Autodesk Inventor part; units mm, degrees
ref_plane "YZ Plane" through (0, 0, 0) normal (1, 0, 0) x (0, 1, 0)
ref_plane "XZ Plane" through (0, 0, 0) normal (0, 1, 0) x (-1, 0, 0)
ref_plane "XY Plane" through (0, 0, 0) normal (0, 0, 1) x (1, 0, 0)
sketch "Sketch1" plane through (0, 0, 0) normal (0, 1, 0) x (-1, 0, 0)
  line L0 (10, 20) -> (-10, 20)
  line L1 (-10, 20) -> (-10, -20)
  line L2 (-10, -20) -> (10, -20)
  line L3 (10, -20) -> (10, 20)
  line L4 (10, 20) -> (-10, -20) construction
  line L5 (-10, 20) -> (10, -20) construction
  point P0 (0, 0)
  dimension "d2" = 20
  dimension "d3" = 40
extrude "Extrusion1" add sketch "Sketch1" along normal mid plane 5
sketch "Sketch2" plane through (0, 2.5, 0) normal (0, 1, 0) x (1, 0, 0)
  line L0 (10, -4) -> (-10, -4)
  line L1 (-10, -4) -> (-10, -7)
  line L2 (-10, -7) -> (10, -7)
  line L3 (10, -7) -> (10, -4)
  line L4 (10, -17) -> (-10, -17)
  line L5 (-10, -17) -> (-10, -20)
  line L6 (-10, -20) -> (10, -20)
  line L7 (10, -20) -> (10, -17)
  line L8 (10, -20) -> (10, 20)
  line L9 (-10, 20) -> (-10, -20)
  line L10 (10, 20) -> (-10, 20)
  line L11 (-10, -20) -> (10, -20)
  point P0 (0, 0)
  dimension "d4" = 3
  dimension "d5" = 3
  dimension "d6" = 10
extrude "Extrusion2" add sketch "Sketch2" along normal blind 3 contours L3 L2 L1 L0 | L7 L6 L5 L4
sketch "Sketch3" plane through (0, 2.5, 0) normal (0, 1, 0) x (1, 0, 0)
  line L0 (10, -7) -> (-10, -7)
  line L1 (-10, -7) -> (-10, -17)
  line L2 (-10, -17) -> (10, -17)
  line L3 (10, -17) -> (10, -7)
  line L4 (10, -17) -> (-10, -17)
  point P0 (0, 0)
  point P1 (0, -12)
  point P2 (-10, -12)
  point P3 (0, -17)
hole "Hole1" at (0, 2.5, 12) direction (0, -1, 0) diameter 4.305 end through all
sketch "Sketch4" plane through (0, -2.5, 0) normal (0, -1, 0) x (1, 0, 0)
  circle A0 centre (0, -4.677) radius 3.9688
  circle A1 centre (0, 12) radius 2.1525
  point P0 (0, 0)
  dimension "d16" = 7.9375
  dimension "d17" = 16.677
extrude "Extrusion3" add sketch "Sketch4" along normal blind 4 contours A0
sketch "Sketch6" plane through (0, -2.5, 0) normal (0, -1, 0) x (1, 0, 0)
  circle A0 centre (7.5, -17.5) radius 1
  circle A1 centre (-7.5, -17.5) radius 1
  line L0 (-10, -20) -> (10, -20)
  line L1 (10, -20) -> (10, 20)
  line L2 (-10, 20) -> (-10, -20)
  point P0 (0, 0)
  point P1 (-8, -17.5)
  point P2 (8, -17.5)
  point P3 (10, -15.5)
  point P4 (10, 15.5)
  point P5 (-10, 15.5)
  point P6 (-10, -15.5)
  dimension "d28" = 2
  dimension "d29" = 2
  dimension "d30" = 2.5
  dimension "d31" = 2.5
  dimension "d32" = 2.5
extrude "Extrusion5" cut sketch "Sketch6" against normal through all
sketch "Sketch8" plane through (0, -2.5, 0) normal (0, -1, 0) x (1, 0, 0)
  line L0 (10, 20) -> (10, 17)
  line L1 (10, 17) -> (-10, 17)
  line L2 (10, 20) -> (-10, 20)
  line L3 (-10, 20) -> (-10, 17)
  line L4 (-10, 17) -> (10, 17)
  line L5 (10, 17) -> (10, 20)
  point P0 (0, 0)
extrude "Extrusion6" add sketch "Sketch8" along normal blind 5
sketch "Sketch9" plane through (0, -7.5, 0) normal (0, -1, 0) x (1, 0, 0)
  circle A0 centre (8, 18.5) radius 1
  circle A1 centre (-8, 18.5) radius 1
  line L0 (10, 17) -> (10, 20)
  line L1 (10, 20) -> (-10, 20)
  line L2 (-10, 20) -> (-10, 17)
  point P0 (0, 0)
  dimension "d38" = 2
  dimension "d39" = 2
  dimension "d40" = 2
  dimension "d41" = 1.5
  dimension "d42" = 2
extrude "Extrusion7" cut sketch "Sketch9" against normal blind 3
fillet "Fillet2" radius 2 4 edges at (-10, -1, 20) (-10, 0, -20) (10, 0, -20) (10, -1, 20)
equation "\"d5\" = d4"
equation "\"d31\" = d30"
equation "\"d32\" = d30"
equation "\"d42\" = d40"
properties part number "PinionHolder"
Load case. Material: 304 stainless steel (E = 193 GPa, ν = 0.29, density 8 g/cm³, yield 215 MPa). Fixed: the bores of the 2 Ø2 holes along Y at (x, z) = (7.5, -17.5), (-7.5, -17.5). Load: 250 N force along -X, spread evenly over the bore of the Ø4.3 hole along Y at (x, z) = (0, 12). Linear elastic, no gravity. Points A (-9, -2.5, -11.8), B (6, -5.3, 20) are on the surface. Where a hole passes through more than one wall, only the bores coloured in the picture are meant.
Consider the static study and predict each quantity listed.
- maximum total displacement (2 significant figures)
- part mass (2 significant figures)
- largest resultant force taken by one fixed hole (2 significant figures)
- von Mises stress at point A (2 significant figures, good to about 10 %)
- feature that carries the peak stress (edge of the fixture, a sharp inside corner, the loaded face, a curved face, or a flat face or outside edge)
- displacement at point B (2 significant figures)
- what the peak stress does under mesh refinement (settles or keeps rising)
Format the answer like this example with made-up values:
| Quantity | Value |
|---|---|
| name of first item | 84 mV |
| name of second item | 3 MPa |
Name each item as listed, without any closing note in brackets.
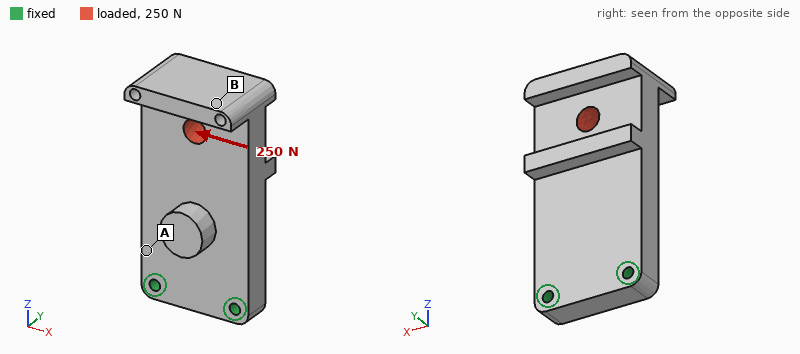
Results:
| Quantity | Value |
|---|---|
| maximum total displacement | 6.2 µm |
| part mass | 38 g |
| largest resultant force taken by one fixed hole | 490 N |
| von Mises stress at point A | 16 MPa |
| feature that carries the peak stress | edge of the fixture |
| displacement at point B | 6.0 µm |
| what the peak stress does under mesh refinement | keeps rising |
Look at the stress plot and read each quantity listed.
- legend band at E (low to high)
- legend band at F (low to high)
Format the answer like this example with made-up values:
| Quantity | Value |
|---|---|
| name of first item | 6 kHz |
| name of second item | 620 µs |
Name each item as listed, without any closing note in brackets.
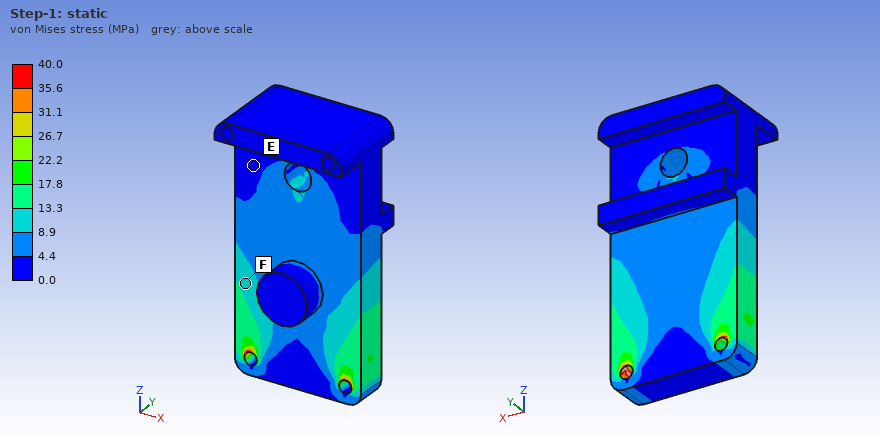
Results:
| Quantity | Value |
|---|---|
| legend band at E | 0.0 to 4.4 MPa |
| legend band at F | 8.9 to 13.3 MPa |
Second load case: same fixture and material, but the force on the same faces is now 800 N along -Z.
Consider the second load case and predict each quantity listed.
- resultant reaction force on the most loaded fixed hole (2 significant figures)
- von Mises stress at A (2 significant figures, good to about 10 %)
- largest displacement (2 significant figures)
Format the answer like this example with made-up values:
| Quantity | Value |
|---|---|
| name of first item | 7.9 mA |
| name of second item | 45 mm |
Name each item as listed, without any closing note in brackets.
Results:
| Quantity | Value |
|---|---|
| resultant reaction force on the most loaded fixed hole | 410 N |
| von Mises stress at A | 10 MPa |
| largest displacement | 1.8 µm |
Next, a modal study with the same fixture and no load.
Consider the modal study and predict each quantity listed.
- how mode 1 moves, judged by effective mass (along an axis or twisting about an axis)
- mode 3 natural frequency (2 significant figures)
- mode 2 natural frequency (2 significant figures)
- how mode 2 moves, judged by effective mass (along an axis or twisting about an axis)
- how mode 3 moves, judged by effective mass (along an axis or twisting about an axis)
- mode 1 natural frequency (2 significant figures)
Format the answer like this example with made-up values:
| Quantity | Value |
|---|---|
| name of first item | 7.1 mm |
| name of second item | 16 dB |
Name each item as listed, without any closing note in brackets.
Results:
| Quantity | Value |
|---|---|
| how mode 1 moves, judged by effective mass | along Y |
| mode 3 natural frequency | 8800 Hz |
| mode 2 natural frequency | 7900 Hz |
| how mode 2 moves, judged by effective mass | along X |
| how mode 3 moves, judged by effective mass | twisting about Z |
| mode 1 natural frequency | 2200 Hz |
